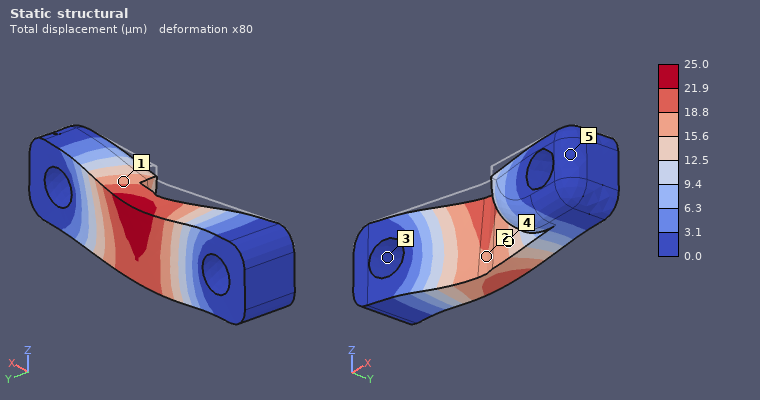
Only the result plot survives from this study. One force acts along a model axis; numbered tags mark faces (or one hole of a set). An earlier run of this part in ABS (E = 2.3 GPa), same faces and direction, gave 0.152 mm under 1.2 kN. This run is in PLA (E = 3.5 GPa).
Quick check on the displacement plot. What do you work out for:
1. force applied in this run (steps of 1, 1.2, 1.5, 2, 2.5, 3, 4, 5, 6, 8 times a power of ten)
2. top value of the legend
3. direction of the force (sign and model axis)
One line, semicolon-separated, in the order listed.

300 N; 25.0 µm; -Z
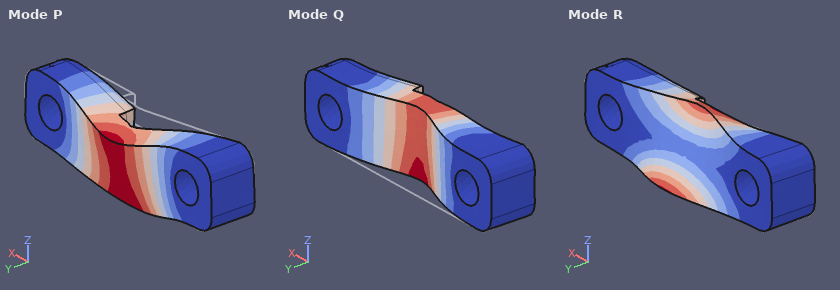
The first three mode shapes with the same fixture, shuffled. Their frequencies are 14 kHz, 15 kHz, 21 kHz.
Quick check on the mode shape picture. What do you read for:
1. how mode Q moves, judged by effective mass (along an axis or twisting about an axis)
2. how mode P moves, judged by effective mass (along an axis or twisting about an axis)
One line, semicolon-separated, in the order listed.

along Y; along Z
